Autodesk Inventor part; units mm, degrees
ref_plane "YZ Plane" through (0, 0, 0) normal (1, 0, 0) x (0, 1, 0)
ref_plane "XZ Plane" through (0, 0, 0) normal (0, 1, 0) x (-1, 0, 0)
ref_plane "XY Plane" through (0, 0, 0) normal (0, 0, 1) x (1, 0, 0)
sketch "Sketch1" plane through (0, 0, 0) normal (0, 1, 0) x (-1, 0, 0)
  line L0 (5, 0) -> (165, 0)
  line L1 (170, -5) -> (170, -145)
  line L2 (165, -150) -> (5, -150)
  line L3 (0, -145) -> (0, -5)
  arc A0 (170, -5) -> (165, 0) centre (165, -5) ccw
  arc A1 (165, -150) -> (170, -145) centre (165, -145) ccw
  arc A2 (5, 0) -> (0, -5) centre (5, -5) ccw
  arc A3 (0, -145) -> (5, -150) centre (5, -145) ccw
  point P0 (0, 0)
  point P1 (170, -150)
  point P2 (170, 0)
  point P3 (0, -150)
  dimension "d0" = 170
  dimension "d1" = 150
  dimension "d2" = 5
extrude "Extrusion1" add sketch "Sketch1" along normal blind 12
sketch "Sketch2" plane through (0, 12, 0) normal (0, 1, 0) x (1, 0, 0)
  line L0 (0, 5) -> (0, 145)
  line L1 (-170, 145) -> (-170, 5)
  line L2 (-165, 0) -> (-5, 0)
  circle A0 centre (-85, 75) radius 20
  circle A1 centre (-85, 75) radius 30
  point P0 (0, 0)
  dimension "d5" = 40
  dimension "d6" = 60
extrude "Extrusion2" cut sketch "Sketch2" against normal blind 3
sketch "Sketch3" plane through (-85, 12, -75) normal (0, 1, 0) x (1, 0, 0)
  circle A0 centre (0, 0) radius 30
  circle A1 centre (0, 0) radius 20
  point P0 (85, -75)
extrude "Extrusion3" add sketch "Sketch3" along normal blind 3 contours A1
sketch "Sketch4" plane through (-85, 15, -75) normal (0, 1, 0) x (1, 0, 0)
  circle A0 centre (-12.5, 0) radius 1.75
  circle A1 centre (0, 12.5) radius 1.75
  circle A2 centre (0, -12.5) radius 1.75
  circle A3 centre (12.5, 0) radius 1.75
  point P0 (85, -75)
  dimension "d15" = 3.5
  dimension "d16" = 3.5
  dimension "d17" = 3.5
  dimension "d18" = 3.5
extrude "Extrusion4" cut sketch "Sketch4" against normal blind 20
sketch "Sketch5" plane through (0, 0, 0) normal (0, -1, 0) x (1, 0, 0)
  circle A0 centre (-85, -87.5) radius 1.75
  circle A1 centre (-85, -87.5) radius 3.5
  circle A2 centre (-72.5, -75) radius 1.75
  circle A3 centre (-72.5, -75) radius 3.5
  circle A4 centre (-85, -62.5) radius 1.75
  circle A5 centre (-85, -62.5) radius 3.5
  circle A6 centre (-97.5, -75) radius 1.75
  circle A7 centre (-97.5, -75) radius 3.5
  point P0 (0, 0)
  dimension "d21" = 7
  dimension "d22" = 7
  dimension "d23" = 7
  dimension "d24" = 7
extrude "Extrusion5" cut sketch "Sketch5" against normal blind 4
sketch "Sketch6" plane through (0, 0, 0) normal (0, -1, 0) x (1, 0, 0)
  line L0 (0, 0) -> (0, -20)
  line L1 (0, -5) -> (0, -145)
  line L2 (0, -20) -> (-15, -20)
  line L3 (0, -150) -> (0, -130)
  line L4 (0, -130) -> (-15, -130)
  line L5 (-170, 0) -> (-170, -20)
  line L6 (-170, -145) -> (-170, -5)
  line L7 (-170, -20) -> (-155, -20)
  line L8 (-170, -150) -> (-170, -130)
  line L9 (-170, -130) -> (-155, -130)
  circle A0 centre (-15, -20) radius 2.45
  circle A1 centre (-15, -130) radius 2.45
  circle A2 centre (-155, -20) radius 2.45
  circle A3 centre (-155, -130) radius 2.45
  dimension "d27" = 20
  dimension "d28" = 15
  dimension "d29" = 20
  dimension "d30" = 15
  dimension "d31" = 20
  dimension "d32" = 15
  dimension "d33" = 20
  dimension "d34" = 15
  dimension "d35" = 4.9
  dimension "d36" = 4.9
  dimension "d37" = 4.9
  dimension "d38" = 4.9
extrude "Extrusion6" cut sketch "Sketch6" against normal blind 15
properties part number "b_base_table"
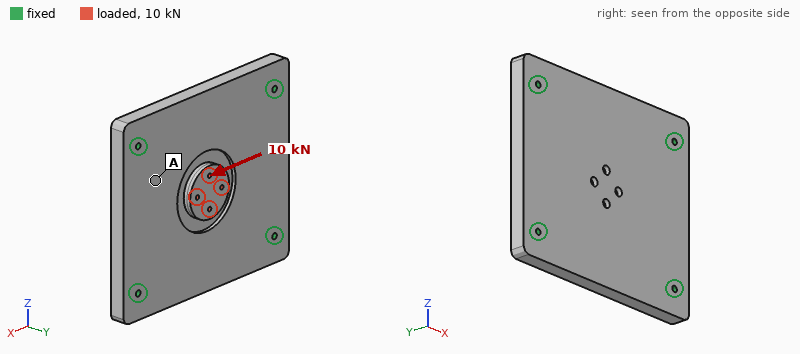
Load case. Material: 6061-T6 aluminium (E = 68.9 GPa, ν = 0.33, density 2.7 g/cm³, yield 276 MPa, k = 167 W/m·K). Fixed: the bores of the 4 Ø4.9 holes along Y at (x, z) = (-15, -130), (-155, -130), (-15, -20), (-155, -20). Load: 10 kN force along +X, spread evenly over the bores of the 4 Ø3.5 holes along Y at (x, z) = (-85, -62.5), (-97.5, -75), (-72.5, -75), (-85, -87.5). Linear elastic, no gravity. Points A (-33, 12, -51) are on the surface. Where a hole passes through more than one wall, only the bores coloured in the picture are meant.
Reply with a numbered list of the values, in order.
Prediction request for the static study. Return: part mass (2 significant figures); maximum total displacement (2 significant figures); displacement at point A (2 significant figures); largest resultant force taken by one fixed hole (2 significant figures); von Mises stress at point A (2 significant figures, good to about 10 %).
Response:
1. 820 g
2. 20 µm
3. 6.7 µm
4. 2.7 kN
5. 3.9 MPa
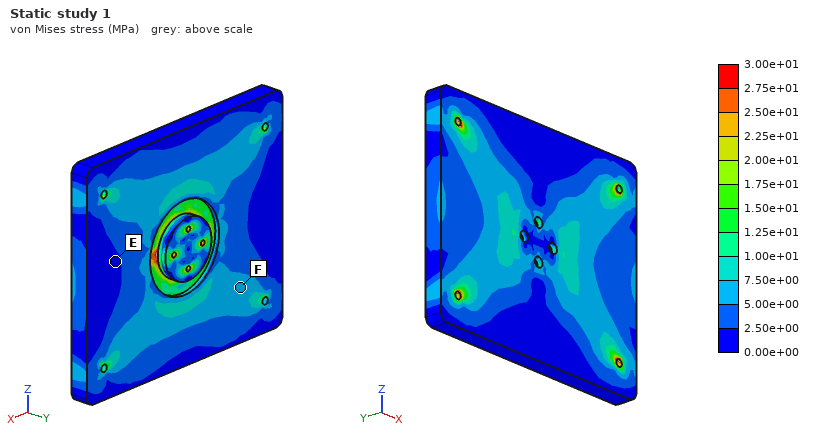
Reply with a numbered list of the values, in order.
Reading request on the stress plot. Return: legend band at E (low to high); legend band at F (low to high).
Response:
1. 0.00e+00 to 2.50e+00 MPa
2. 5.00e+00 to 7.50e+00 MPa
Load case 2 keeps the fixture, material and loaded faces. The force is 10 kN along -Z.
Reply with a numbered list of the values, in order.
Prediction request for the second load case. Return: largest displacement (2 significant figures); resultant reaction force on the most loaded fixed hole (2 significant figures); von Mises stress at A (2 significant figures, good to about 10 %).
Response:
1. 23 µm
2. 2.8 kN
3. 8.0 MPa
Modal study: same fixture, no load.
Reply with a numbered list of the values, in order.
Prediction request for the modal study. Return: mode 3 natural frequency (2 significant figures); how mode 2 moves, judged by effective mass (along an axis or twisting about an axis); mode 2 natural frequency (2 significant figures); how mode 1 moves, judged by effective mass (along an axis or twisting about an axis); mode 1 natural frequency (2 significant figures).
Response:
1. 3900 Hz
2. twisting about X
3. 3100 Hz
4. along Y
5. 2100 Hz
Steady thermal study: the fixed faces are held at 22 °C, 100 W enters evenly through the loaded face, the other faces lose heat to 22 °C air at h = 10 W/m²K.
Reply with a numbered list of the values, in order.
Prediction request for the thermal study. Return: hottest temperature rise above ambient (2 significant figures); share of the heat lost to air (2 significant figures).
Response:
1. 26 K
2. 5.3 %
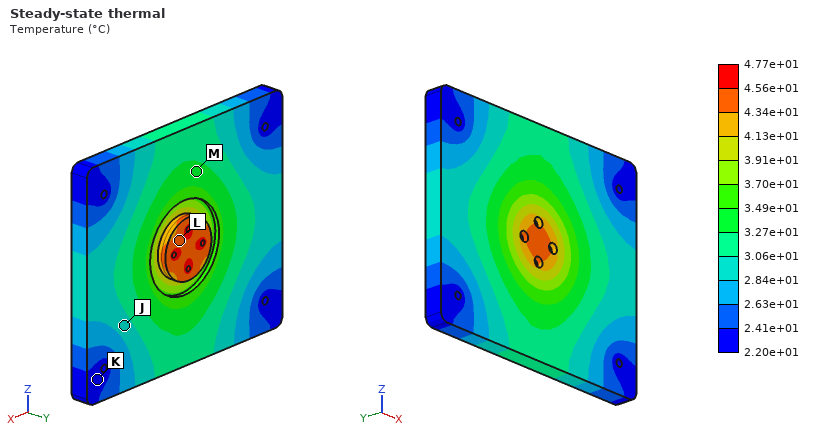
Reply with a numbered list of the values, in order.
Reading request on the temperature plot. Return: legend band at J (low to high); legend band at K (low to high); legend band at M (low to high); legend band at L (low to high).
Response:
1. 2.84e+01 to 3.06e+01 °C
2. 2.20e+01 to 2.41e+01 °C
3. 3.27e+01 to 3.49e+01 °C
4. 4.34e+01 to 4.56e+01 °C
